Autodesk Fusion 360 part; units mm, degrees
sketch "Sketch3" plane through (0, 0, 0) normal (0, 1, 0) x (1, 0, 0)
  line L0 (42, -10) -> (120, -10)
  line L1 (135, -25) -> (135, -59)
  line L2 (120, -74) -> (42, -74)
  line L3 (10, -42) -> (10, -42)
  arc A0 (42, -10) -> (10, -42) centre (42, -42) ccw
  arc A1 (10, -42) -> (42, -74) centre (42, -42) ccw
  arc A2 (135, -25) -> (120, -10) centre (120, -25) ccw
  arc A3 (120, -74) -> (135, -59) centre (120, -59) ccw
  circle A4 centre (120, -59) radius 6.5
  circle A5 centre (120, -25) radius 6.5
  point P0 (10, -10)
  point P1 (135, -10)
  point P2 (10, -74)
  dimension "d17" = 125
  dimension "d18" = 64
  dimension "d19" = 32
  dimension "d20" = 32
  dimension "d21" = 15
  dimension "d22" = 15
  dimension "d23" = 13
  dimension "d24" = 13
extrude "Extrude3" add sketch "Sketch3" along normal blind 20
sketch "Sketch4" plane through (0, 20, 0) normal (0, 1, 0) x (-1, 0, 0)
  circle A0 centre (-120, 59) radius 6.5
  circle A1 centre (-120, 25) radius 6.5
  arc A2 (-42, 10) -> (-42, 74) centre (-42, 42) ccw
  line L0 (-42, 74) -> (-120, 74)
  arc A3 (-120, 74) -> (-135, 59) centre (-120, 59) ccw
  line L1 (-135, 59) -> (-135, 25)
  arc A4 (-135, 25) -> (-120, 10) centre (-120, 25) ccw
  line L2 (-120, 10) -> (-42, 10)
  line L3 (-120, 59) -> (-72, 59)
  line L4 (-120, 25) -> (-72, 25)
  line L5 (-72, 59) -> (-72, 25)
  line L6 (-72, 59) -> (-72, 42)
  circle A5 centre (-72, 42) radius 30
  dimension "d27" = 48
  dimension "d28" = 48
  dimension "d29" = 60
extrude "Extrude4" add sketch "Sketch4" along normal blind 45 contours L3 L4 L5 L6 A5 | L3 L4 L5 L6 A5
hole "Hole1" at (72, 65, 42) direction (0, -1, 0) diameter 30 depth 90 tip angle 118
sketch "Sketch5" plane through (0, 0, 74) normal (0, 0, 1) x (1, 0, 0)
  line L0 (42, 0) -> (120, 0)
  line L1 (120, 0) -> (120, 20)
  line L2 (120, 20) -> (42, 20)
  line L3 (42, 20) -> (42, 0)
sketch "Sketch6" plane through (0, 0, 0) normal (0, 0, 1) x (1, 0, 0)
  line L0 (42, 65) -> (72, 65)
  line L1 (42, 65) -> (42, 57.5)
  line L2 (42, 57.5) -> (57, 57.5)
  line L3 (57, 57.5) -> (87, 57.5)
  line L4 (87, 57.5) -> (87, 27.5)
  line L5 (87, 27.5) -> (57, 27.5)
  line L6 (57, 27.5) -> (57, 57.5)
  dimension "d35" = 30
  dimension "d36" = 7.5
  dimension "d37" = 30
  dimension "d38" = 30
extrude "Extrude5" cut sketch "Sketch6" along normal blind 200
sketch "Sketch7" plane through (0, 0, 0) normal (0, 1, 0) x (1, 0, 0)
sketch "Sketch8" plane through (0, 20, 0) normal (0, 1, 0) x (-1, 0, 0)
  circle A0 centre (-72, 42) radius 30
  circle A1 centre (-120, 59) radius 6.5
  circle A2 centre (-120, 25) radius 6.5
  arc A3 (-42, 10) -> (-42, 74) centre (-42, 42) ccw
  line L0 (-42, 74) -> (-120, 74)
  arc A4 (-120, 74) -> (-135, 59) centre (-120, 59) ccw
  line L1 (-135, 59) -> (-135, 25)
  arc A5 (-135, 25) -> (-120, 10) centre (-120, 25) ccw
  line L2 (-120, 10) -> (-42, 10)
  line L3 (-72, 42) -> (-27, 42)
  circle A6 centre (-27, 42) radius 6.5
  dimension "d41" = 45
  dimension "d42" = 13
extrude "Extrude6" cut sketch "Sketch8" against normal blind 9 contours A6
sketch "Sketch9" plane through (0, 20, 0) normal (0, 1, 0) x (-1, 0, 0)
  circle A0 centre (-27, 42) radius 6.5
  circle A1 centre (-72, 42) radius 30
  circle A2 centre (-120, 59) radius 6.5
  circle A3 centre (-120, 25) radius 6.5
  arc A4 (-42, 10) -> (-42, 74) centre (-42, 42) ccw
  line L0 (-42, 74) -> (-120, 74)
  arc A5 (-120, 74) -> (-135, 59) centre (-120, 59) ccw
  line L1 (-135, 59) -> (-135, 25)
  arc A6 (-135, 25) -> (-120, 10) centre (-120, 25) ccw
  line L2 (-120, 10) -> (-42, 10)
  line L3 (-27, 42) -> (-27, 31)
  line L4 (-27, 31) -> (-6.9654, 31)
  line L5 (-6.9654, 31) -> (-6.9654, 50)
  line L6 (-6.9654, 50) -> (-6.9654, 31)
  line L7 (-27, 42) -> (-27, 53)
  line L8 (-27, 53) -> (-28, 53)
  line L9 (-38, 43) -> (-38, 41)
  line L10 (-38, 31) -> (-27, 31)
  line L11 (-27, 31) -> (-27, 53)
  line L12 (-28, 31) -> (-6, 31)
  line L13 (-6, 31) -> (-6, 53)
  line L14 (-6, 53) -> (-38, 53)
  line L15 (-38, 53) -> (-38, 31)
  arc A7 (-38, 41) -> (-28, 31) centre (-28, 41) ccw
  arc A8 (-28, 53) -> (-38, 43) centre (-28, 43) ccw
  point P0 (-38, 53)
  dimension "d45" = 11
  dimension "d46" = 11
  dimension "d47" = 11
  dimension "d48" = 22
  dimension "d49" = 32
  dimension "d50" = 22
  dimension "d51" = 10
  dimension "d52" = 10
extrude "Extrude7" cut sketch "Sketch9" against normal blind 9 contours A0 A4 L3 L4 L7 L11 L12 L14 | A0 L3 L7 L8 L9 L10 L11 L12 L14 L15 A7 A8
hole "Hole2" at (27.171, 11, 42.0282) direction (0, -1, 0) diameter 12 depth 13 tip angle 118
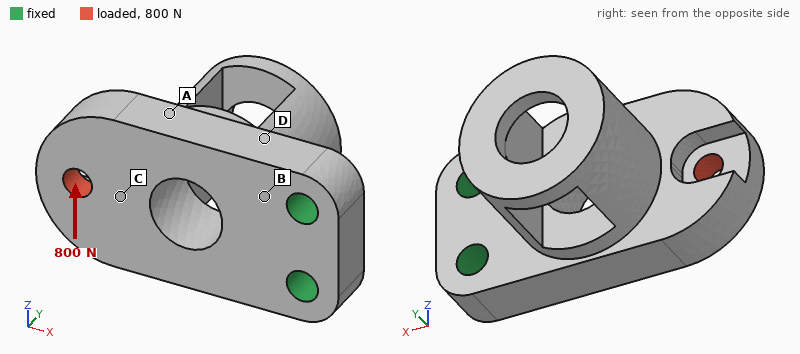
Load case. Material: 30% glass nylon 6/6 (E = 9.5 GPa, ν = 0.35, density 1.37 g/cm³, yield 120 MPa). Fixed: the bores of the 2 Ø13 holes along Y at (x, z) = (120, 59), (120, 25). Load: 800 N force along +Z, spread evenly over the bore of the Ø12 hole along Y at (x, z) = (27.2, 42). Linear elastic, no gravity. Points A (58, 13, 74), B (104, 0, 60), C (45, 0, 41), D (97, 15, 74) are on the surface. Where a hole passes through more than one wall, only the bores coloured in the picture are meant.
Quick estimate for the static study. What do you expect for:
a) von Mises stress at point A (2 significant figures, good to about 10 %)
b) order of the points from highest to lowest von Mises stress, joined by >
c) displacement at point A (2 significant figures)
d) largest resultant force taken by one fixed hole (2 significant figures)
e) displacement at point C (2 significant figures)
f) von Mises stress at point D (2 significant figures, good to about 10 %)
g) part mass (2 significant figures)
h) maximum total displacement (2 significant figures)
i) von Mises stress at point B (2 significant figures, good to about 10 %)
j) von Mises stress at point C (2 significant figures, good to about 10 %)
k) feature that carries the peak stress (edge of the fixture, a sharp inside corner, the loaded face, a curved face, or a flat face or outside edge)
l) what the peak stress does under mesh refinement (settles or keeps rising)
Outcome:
0.93 MPa
D > C > B > A
0.064 mm
1.7 kN
0.077 mm
5.3 MPa
260 g
0.11 mm
2.0 MPa
4.0 MPa
edge of the fixture
keeps rising
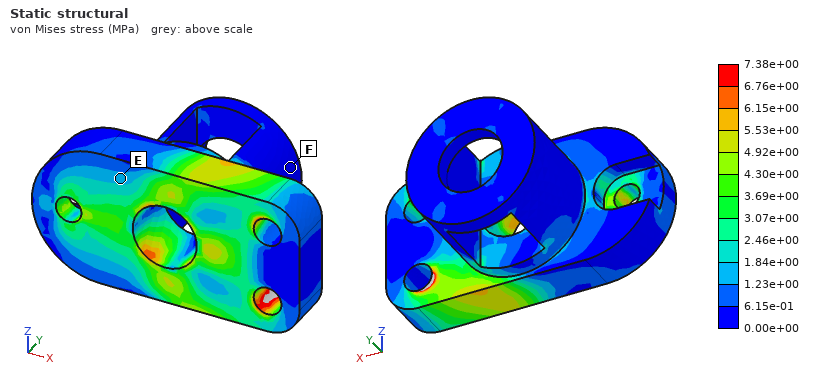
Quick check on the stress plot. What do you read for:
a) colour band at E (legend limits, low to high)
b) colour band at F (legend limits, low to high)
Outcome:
1.23e+00 to 1.84e+00 MPa
0.00e+00 to 6.15e-01 MPa
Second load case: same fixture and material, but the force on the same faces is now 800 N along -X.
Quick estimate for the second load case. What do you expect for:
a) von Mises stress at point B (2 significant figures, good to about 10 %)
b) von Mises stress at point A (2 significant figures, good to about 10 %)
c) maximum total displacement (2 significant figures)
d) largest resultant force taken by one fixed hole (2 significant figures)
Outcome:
1.7 MPa
0.33 MPa
59 µm
400 N
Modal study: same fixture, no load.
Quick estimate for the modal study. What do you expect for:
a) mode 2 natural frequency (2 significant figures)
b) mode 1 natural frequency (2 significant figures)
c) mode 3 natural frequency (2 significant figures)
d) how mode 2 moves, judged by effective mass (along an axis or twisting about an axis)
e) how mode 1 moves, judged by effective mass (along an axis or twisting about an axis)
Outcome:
1600 Hz
740 Hz
1900 Hz
along Z
along Y
